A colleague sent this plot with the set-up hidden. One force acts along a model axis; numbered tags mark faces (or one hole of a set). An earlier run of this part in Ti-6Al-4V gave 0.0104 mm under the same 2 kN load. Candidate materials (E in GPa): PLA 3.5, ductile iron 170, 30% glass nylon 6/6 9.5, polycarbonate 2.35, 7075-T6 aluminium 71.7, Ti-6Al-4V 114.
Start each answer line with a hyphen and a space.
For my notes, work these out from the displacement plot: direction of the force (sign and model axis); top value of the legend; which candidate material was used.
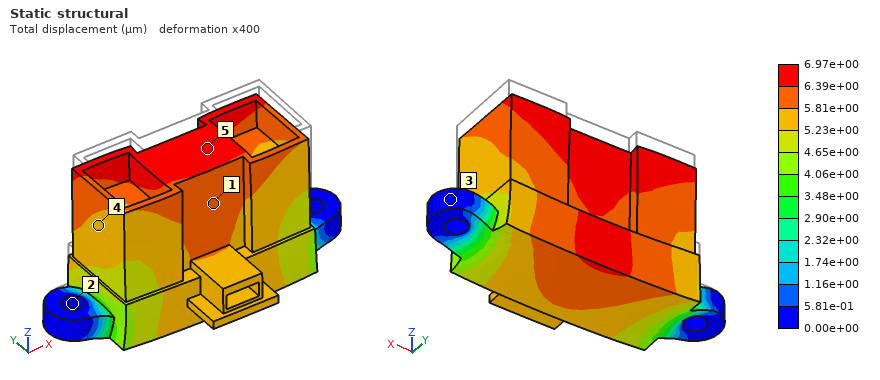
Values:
- -Z
- 6.97e+00 µm
- ductile iron
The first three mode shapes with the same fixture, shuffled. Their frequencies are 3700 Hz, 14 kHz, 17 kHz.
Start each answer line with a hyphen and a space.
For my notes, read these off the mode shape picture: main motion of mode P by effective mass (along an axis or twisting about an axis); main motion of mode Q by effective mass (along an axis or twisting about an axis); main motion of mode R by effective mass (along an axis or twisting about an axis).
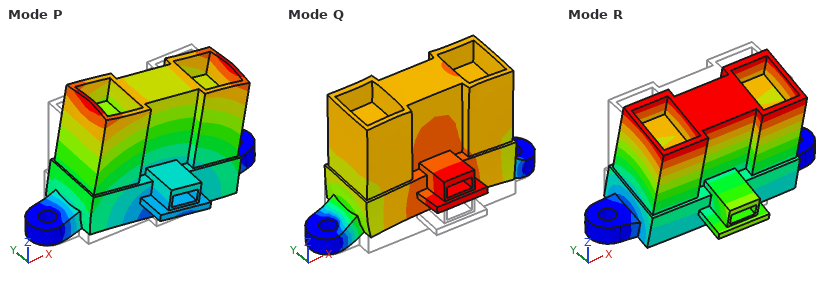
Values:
- along X
- along Z
- along Y
